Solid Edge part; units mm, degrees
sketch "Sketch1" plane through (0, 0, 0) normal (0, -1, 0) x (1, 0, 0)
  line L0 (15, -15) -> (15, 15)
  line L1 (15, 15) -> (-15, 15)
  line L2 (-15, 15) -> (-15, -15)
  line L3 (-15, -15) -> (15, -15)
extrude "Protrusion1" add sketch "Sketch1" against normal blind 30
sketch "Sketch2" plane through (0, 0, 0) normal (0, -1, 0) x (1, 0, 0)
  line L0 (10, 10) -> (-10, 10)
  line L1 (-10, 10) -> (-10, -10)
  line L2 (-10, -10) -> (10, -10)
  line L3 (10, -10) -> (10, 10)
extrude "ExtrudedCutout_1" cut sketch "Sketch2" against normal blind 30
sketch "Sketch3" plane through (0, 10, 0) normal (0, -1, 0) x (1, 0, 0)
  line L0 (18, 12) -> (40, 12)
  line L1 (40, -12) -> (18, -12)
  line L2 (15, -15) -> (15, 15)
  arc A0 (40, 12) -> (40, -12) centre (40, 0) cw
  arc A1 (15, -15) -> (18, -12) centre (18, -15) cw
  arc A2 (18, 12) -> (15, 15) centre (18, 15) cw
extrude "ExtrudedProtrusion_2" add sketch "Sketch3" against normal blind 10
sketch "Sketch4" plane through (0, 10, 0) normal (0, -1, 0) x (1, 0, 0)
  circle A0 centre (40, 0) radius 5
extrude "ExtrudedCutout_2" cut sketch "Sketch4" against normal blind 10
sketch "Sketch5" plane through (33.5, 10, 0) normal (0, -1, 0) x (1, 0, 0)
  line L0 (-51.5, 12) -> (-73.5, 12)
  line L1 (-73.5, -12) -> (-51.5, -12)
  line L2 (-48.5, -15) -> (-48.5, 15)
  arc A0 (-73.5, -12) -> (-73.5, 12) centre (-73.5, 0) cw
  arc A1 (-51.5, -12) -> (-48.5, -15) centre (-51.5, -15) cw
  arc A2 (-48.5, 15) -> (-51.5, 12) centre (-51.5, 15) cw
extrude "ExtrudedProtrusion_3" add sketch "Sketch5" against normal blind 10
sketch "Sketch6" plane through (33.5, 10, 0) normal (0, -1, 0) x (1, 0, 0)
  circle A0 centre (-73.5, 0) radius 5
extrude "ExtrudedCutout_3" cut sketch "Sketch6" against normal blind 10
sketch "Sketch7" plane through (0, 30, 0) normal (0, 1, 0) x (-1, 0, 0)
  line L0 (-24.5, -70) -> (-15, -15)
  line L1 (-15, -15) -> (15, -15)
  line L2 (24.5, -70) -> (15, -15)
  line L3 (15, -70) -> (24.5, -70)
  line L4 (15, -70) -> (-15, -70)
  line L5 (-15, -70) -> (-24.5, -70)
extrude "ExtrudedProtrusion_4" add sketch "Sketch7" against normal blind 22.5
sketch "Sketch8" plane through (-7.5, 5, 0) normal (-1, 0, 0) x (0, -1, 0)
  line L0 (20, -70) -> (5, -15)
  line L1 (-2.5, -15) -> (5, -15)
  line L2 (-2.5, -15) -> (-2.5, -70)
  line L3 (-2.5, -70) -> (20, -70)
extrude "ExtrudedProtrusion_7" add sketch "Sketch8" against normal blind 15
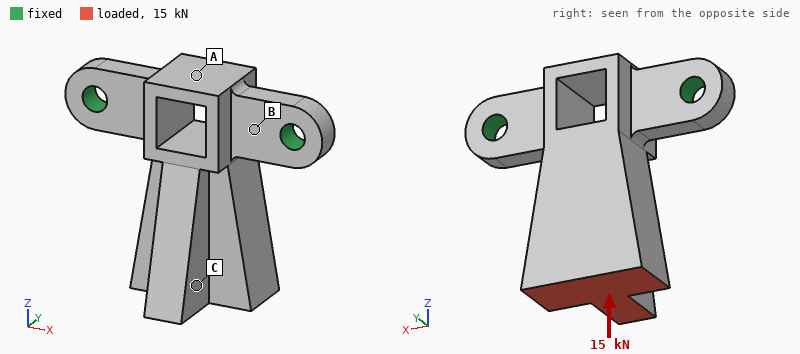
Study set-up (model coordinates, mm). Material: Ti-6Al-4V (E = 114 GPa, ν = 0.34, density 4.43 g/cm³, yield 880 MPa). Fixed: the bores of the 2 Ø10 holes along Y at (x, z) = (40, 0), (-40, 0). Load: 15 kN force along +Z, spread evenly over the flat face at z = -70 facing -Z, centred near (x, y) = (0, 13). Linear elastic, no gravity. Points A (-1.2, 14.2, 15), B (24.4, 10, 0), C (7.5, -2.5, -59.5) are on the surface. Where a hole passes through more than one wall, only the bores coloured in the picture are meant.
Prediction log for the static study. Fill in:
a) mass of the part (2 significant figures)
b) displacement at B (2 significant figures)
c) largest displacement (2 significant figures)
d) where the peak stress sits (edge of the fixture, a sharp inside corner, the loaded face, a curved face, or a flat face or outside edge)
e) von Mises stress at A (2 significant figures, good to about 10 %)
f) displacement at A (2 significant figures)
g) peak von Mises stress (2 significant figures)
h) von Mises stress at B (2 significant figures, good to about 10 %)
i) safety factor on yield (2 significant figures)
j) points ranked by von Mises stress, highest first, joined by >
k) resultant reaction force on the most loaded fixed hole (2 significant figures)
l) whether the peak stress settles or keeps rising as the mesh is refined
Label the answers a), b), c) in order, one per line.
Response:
a) 400 g
b) 0.022 mm
c) 0.13 mm
d) a curved face
e) 43 MPa
f) 0.035 mm
g) 270 MPa
h) 100 MPa
i) 3.3
j) B > A > C
k) 7.7 kN
l) settles
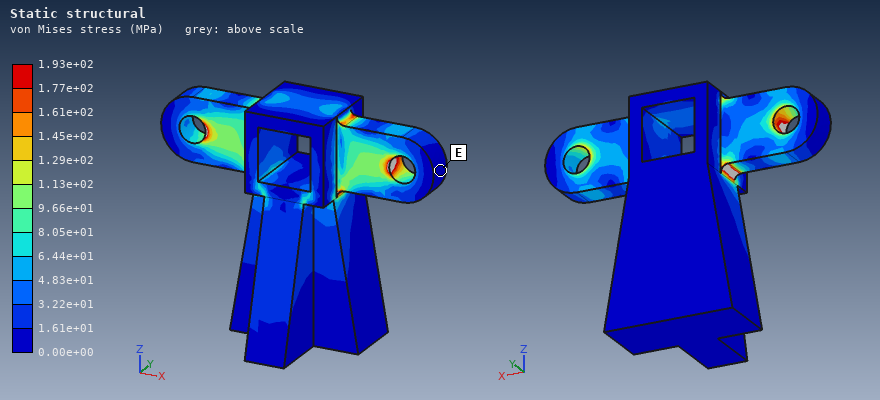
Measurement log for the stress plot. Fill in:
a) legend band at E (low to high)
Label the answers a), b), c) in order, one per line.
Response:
a) 0.00e+00 to 1.61e+01 MPa
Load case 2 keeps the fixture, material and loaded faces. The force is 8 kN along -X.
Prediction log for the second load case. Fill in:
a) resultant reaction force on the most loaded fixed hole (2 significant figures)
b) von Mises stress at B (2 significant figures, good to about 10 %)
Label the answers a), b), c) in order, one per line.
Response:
a) 12 kN
b) 100 MPa
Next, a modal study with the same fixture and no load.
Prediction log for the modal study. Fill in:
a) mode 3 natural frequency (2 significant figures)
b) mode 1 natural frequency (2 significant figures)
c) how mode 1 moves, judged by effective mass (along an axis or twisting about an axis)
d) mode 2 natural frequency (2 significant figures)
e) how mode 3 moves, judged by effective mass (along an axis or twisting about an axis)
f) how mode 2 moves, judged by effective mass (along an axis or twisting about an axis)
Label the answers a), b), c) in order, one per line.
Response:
a) 4900 Hz
b) 890 Hz
c) along Y
d) 2100 Hz
e) twisting about Z
f) along X
